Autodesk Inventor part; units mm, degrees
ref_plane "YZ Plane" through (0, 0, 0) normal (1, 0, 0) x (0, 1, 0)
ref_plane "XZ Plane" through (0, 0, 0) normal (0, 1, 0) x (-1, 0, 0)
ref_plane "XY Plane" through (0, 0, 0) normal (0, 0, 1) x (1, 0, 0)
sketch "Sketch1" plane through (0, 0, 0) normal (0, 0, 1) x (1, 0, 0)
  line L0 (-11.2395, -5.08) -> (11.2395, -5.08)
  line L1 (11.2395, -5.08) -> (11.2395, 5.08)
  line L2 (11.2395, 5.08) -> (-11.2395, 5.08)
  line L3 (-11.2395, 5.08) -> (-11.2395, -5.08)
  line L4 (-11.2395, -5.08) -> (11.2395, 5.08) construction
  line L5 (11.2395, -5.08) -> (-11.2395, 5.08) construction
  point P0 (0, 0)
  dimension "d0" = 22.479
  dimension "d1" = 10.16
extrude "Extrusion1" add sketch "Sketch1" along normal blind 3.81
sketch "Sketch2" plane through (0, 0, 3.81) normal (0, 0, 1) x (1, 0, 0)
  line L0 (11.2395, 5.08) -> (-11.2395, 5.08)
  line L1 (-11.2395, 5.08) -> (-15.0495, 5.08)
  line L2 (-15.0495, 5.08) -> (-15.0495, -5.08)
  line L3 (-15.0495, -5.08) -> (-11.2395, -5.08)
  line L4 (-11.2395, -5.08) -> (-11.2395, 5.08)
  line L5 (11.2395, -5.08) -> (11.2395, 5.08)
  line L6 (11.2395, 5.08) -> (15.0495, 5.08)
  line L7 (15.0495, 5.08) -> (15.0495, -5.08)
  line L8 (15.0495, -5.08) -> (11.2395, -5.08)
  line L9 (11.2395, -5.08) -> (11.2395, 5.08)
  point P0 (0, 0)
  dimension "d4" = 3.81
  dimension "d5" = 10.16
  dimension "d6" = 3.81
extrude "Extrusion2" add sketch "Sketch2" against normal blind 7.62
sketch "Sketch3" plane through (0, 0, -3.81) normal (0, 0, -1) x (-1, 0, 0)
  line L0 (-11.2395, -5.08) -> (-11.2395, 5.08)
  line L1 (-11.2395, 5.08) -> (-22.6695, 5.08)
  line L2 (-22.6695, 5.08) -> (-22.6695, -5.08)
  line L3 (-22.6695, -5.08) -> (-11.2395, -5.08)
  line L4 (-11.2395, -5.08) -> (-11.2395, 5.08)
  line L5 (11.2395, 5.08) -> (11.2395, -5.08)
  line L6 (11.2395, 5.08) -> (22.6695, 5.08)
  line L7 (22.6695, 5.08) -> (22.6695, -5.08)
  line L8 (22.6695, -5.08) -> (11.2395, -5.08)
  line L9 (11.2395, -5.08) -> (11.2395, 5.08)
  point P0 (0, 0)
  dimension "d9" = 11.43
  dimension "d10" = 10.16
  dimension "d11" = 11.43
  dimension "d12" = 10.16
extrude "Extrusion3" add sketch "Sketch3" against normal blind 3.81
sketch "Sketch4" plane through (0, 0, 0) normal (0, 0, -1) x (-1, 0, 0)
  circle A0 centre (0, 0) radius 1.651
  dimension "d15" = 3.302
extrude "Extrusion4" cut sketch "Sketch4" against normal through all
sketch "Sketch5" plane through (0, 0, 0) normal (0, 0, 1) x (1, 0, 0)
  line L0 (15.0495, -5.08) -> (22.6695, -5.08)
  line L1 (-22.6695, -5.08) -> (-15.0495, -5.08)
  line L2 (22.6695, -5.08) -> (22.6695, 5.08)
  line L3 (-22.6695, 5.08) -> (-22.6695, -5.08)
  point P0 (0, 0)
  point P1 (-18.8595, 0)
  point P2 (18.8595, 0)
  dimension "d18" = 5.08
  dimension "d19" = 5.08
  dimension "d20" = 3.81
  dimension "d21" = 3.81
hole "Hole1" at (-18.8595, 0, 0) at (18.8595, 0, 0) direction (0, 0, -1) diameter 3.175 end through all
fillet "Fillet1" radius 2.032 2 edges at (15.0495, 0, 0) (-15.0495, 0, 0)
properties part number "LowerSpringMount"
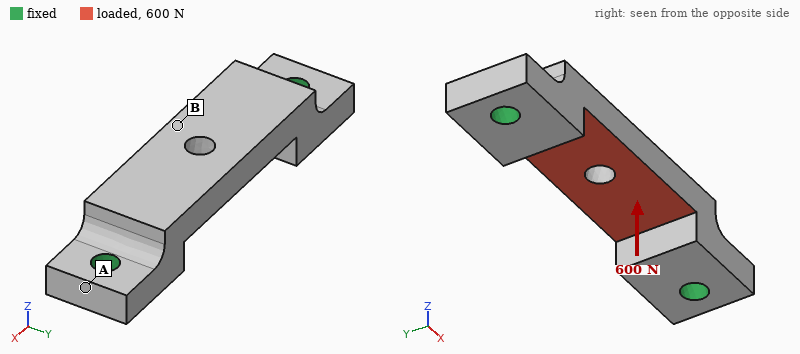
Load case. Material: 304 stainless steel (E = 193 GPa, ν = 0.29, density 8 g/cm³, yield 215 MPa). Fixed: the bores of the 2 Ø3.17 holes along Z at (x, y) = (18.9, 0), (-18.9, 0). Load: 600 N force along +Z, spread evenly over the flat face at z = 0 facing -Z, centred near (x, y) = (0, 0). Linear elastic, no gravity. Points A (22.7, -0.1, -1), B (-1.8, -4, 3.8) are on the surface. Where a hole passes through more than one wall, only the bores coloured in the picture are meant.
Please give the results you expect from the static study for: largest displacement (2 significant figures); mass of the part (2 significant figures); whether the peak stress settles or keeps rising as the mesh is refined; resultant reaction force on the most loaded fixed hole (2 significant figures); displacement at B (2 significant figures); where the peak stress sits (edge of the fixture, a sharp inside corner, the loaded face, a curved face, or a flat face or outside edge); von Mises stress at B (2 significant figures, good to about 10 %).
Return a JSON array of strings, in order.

["8.4 µm", "16 g", "keeps rising", "550 N", "8.0 µm", "edge of the fixture", "58 MPa"]
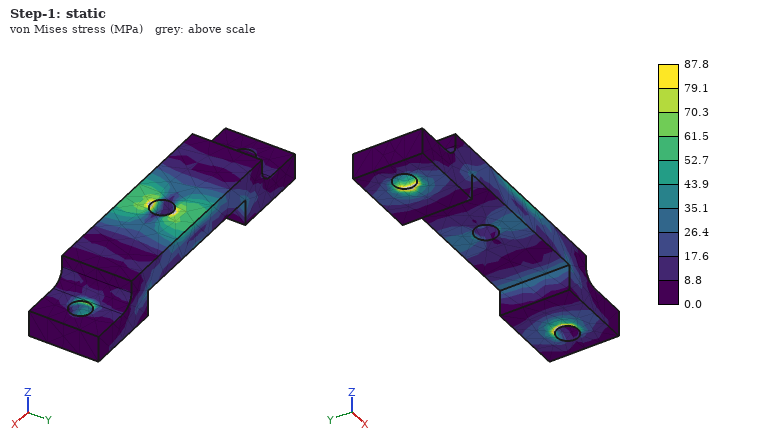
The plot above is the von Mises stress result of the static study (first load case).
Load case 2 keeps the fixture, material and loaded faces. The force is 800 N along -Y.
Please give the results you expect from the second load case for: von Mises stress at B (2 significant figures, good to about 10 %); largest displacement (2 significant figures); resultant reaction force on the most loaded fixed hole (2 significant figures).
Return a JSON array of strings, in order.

["38 MPa", "7.4 µm", "400 N"]
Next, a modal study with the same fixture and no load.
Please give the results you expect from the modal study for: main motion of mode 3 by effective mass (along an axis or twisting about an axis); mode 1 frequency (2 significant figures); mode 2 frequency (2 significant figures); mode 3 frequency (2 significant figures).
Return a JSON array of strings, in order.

["along X", "18 kHz", "19 kHz", "27 kHz"]
